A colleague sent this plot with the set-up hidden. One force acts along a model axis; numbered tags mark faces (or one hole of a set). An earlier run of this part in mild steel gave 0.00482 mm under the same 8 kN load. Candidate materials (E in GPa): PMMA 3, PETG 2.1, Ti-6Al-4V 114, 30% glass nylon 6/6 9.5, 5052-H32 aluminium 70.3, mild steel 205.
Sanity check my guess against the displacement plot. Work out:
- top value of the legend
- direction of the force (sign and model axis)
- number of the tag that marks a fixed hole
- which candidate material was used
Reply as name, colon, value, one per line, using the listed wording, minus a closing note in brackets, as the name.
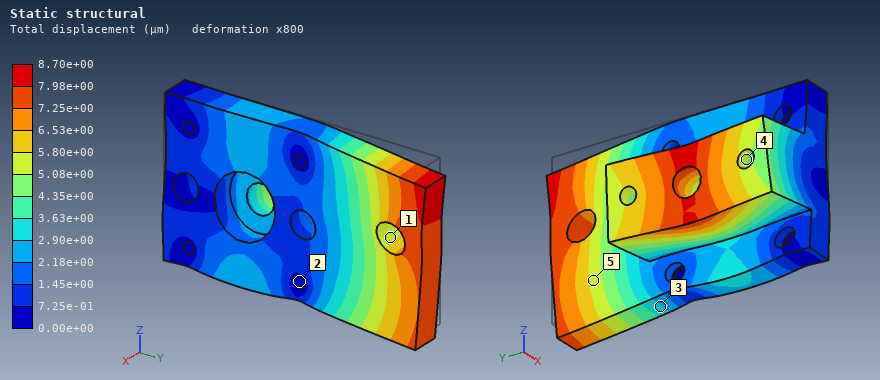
top value of the legend: 8.70e+00 µm
direction of the force: -Z
number of the tag that marks a fixed hole: 2
which candidate material was used: Ti-6Al-4V
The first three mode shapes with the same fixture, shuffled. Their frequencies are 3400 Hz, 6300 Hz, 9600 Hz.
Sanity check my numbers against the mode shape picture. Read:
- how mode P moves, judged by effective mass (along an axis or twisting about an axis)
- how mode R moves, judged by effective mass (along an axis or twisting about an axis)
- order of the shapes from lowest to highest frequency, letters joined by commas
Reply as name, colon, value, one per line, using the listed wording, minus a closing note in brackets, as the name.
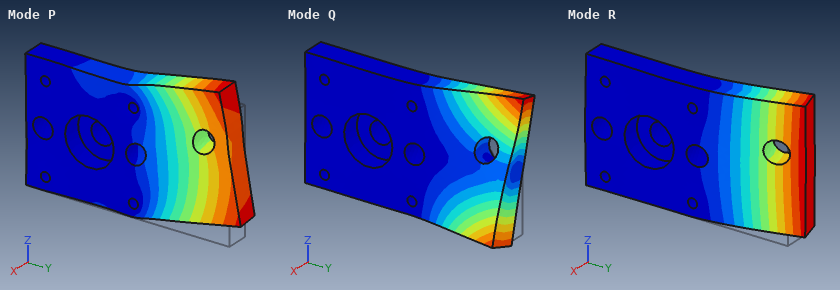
how mode P moves, judged by effective mass: along Z
how mode R moves, judged by effective mass: along X
order of the shapes from lowest to highest frequency, letters joined by commas: R, Q, P
